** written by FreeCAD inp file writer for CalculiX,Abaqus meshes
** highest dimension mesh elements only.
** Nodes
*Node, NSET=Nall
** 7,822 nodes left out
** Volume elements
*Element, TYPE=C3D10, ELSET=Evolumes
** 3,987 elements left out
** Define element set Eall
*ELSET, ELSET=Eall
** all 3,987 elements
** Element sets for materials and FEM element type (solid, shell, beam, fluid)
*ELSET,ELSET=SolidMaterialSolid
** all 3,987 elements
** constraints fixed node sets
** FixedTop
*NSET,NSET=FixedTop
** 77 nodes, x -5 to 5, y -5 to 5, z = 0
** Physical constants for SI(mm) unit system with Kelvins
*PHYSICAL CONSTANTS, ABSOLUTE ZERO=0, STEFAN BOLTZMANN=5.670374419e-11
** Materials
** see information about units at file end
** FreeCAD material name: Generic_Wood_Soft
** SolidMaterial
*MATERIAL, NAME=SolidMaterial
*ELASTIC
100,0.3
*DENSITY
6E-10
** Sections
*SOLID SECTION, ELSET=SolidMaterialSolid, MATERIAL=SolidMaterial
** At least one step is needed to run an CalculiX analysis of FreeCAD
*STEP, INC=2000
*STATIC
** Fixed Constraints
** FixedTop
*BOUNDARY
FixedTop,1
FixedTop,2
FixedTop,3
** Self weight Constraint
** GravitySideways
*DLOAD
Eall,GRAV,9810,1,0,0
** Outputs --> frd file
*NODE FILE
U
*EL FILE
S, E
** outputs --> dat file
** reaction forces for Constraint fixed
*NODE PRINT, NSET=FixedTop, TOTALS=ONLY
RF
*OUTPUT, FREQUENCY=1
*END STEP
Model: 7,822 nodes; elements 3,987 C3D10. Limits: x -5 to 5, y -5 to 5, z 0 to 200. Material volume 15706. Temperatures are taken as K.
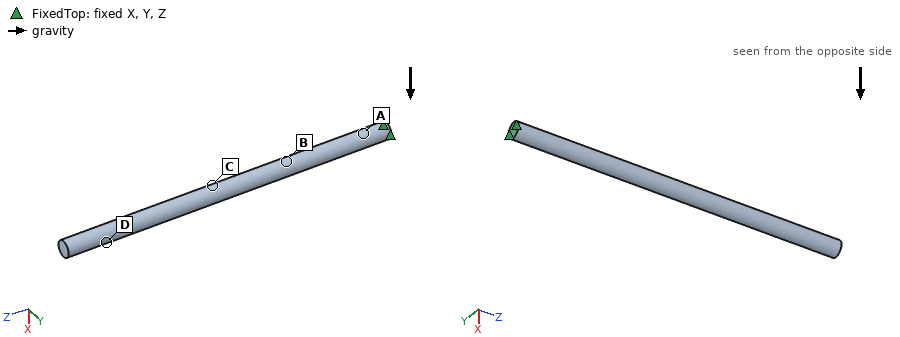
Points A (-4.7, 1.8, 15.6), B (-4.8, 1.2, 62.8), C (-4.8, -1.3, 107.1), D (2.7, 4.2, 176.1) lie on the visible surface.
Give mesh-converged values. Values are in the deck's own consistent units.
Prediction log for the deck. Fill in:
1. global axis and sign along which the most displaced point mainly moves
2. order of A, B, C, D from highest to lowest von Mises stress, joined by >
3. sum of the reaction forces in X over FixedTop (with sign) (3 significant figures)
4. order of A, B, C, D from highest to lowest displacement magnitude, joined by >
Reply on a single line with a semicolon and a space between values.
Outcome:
+X; A > B > C > D; -0.0924; D > C > B > A
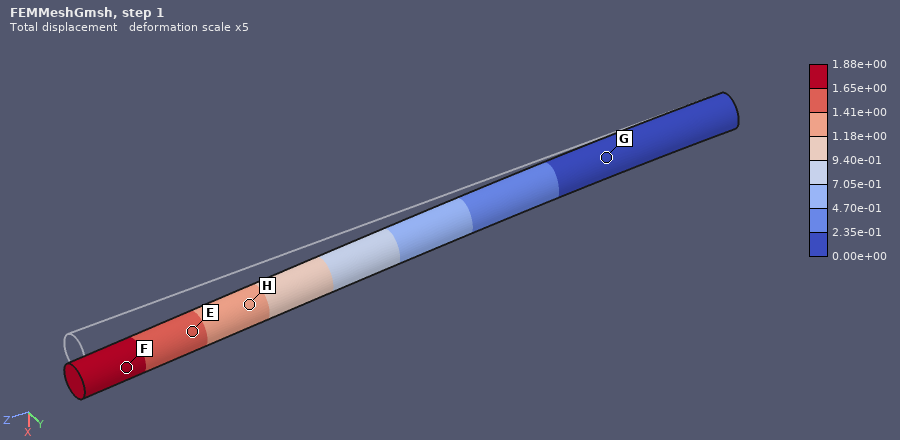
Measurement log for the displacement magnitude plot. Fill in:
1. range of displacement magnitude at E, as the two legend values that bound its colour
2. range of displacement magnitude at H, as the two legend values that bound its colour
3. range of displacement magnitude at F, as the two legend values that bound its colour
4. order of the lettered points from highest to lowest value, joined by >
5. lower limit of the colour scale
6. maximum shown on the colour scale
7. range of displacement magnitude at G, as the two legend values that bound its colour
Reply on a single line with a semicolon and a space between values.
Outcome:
1.41e+00 to 1.65e+00; 1.18e+00 to 1.41e+00; 1.65e+00 to 1.88e+00; F > E > H > G; 0.00e+00; 1.88e+00; 0.00e+00 to 2.35e-01
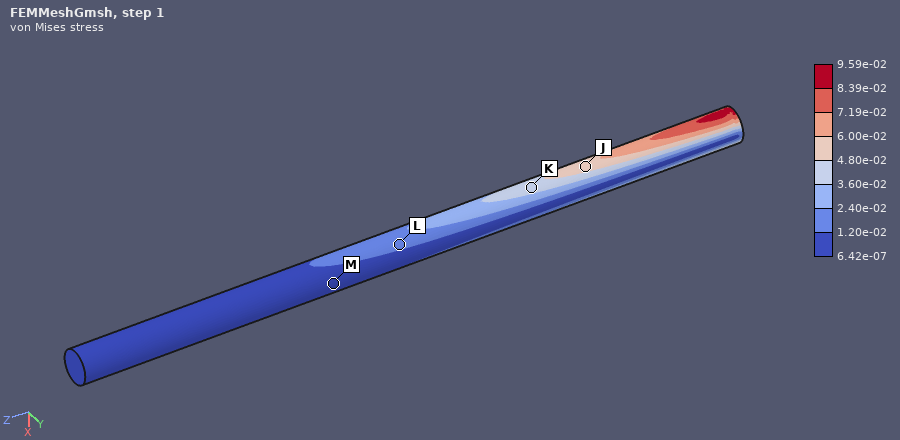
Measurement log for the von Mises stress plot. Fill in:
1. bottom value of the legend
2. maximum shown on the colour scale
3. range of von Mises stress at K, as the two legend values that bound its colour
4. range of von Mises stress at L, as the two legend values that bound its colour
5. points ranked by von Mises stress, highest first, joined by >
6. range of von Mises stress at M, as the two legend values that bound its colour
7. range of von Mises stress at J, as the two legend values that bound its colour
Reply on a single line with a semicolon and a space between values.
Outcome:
6.42e-07; 9.59e-02; 3.60e-02 to 4.80e-02; 1.20e-02 to 2.40e-02; J > K > L > M; 6.42e-07 to 1.20e-02; 4.80e-02 to 6.00e-02
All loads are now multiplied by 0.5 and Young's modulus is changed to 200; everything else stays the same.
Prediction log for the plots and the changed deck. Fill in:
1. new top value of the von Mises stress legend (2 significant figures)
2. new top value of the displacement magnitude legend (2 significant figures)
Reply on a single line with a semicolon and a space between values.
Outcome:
0.048; 0.47
